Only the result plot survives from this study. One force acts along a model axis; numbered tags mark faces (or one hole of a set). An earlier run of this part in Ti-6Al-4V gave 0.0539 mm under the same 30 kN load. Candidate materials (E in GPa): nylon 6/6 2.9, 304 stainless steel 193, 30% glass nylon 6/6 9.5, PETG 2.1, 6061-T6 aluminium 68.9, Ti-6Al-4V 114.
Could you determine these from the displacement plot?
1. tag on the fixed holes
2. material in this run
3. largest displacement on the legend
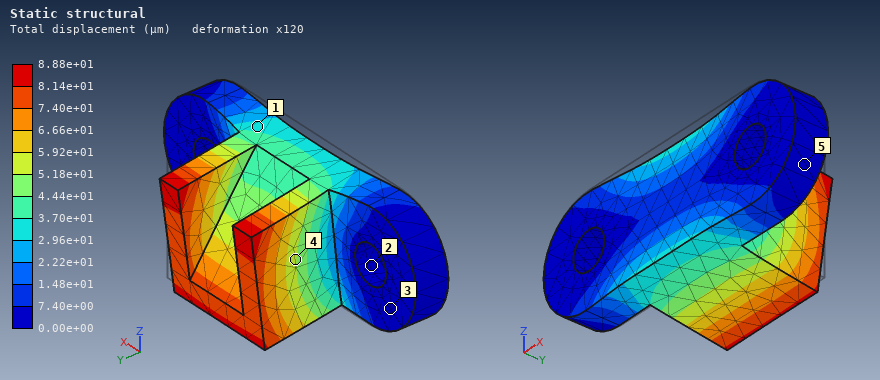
2
6061-T6 aluminium
8.88e+01 µm
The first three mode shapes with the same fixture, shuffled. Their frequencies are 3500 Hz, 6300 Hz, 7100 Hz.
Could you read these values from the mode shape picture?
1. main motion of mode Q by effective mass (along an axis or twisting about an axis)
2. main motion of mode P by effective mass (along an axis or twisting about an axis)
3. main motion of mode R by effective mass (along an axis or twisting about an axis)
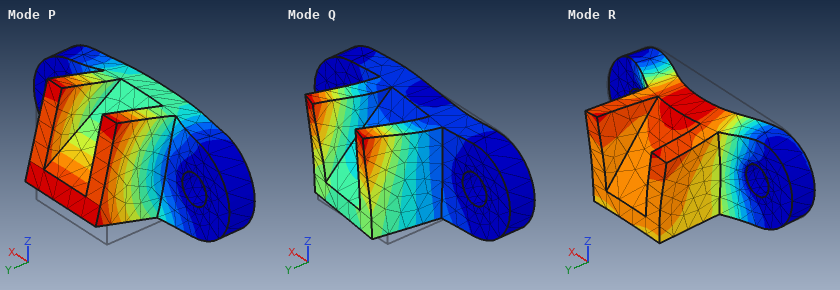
along X
along Z
along Y
